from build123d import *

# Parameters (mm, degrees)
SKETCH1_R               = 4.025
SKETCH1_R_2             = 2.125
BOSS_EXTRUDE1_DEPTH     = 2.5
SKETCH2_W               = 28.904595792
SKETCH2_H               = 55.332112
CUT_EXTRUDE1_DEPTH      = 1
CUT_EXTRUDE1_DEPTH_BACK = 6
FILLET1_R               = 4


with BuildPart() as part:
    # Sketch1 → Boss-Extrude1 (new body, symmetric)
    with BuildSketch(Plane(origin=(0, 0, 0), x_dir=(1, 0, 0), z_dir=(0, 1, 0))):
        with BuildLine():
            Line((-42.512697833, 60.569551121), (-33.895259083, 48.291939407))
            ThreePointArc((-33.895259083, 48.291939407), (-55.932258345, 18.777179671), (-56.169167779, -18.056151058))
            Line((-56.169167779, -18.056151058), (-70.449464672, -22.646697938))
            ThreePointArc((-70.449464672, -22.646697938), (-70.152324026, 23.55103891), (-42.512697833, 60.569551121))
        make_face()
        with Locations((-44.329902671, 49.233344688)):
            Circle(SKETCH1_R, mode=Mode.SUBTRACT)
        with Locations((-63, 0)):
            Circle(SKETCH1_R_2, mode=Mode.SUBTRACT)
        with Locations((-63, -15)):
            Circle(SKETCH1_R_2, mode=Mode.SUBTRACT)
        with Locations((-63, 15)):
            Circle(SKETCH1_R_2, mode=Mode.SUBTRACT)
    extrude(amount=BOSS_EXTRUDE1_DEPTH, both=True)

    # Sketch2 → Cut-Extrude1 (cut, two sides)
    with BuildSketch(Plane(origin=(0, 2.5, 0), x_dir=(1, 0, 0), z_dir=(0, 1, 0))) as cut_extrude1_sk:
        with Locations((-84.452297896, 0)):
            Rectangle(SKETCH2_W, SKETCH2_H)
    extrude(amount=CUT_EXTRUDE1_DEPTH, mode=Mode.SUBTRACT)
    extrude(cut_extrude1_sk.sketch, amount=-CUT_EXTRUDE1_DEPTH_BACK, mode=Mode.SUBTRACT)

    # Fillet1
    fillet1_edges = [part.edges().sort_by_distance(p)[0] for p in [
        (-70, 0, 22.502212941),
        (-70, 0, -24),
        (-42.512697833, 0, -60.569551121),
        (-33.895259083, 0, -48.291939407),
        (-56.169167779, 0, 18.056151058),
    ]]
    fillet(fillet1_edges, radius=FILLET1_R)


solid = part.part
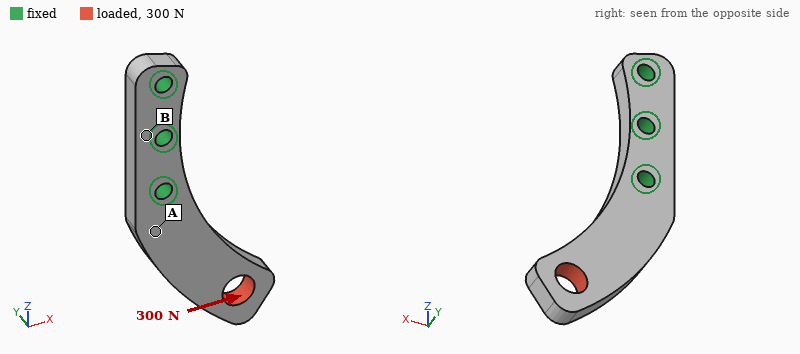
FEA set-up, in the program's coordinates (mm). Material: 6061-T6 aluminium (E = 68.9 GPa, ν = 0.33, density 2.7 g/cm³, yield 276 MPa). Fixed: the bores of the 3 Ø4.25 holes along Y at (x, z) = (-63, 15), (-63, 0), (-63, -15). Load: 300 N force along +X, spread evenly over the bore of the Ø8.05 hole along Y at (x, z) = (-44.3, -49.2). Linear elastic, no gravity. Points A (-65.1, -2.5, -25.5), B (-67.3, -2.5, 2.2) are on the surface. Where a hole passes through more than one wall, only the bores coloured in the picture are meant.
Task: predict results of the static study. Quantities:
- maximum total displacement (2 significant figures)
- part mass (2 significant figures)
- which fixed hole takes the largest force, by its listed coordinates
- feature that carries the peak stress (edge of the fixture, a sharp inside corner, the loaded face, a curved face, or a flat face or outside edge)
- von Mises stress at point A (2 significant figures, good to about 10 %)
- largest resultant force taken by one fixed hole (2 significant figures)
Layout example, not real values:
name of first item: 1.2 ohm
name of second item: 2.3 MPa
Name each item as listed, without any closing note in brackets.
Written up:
maximum total displacement: 0.12 mm
part mass: 14 g
which fixed hole takes the largest force, by its listed coordinates: (-63, -15)
feature that carries the peak stress: edge of the fixture
von Mises stress at point A: 24 MPa
largest resultant force taken by one fixed hole: 610 N
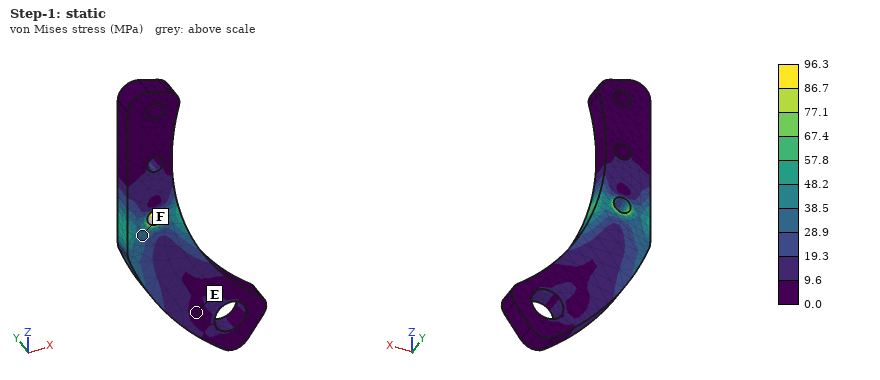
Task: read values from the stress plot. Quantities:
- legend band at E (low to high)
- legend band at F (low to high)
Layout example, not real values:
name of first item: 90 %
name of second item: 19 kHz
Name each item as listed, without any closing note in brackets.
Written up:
legend band at E: 0.0 to 9.6 MPa
legend band at F: 28.9 to 38.5 MPa
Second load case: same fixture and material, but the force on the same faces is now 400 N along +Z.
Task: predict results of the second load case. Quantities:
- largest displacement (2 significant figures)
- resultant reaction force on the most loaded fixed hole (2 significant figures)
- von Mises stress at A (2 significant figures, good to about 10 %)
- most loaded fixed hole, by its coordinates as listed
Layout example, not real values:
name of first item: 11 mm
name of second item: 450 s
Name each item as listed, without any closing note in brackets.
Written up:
largest displacement: 0.10 mm
resultant reaction force on the most loaded fixed hole: 510 N
von Mises stress at A: 15 MPa
most loaded fixed hole, by its coordinates as listed: (-63, -15)
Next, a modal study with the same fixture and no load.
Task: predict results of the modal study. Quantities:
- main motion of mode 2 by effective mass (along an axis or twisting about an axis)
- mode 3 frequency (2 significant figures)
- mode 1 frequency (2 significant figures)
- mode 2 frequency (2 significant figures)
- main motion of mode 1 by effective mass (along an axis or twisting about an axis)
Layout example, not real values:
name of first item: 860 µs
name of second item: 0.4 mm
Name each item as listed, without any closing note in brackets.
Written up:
main motion of mode 2 by effective mass: along X
mode 3 frequency: 8500 Hz
mode 1 frequency: 2000 Hz
mode 2 frequency: 4400 Hz
main motion of mode 1 by effective mass: along Y
